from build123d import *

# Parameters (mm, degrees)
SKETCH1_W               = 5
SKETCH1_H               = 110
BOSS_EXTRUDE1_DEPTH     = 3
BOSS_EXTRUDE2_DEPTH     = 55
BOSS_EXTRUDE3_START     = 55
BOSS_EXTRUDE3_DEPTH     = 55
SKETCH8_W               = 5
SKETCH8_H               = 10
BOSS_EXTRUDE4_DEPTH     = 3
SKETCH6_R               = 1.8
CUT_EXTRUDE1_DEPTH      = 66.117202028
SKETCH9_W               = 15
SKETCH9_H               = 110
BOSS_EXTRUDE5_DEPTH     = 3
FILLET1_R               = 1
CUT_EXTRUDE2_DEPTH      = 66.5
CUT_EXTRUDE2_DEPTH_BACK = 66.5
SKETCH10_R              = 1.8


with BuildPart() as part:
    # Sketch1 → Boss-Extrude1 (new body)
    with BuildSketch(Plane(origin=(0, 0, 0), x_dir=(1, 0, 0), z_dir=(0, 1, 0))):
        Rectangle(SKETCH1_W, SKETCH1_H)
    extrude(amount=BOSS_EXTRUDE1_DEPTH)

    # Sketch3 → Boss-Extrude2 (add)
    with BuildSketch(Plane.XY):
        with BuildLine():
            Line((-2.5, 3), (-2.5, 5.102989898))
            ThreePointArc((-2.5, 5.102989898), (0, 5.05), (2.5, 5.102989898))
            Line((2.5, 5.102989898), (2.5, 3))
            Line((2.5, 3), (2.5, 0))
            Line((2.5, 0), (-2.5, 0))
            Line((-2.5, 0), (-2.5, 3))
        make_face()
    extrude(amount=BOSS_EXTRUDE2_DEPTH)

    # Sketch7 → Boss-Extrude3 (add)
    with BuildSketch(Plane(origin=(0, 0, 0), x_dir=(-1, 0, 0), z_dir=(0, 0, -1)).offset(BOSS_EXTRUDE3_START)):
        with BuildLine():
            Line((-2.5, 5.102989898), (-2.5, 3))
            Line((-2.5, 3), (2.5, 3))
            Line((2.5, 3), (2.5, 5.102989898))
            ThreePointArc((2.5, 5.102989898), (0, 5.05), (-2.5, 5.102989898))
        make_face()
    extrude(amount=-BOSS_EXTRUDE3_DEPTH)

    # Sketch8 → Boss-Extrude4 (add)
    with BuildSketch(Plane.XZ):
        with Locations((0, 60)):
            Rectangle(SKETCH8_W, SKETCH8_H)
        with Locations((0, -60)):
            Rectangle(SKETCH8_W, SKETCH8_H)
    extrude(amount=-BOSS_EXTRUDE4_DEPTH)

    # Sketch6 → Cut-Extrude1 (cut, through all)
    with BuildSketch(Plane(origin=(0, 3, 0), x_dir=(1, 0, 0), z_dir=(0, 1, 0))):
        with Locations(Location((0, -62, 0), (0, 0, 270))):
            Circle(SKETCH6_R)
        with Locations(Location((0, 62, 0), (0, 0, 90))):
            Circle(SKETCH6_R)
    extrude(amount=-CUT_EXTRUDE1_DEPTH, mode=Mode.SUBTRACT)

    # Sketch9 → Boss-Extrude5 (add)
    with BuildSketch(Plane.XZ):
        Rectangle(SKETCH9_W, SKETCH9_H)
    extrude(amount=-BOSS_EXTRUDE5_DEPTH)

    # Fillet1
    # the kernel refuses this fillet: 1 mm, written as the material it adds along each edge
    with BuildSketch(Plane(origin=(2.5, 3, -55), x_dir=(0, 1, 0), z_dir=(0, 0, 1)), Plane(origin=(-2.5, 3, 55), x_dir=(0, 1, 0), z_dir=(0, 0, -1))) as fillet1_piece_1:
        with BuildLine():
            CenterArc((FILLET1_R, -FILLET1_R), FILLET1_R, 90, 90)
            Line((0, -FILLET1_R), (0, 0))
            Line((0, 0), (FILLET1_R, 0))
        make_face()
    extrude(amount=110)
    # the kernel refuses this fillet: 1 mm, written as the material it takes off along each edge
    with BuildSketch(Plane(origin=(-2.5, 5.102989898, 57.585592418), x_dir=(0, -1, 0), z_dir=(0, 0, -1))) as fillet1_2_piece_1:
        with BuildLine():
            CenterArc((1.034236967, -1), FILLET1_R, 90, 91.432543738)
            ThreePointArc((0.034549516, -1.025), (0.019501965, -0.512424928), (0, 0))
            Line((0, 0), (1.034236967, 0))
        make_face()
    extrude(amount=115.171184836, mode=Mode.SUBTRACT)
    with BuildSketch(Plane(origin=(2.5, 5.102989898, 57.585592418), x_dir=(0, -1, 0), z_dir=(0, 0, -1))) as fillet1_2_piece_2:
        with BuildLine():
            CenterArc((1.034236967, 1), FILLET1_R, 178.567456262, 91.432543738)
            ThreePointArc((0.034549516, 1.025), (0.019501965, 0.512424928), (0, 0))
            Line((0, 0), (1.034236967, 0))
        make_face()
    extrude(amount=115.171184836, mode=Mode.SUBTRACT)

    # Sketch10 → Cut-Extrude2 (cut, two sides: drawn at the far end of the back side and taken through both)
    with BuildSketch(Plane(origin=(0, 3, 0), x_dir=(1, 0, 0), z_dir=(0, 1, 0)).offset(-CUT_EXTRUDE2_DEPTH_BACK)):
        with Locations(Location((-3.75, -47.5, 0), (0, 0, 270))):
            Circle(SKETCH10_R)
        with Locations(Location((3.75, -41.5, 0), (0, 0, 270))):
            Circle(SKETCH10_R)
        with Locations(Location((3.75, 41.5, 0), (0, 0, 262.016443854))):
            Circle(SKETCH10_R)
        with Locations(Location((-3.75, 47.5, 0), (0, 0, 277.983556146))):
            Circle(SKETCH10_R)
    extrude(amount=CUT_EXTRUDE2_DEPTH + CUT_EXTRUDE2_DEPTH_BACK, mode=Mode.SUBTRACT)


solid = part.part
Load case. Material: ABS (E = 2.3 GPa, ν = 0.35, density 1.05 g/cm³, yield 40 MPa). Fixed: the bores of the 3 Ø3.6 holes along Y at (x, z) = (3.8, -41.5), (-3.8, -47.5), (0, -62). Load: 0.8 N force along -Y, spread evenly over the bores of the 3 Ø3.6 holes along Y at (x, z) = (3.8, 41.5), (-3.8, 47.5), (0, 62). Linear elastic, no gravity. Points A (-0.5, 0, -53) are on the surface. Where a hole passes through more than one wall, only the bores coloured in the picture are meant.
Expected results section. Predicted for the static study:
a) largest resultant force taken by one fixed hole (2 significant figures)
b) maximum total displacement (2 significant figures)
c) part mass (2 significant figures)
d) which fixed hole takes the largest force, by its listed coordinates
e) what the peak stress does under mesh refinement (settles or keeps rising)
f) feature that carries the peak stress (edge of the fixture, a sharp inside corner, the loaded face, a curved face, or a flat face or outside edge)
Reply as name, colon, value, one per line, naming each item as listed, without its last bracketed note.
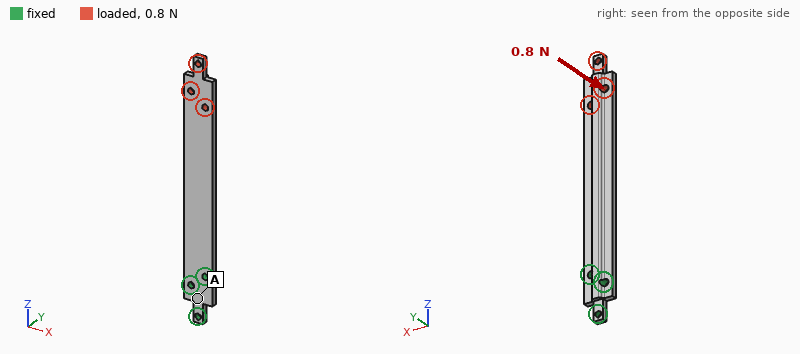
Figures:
largest resultant force taken by one fixed hole: 4.1 N
maximum total displacement: 1.3 mm
part mass: 6.5 g
which fixed hole takes the largest force, by its listed coordinates: (3.8, -41.5)
what the peak stress does under mesh refinement: keeps rising
feature that carries the peak stress: edge of the fixture
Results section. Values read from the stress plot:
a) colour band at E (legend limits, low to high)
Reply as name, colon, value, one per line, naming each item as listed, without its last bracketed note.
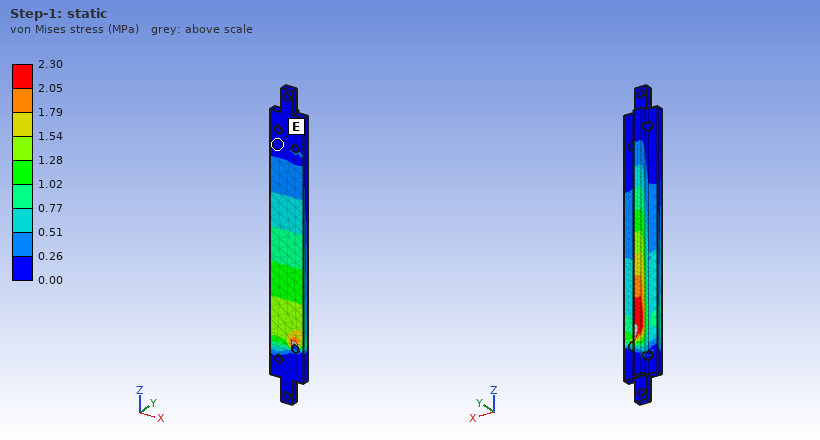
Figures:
colour band at E: 0.00 to 0.26 MPa
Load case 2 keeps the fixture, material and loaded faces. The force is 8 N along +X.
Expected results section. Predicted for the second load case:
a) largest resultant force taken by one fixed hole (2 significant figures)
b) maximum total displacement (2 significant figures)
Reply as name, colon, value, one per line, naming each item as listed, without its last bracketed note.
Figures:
largest resultant force taken by one fixed hole: 69 N
maximum total displacement: 1.4 mm
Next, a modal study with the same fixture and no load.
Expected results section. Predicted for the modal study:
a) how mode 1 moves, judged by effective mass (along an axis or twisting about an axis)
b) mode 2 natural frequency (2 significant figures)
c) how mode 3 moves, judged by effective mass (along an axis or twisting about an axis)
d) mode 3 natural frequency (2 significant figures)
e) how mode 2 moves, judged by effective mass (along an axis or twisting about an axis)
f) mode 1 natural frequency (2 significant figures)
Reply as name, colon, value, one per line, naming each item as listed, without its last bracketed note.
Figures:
how mode 1 moves, judged by effective mass: along Y
mode 2 natural frequency: 320 Hz
how mode 3 moves, judged by effective mass: along Y
mode 3 natural frequency: 650 Hz
how mode 2 moves, judged by effective mass: along X
mode 1 natural frequency: 110 Hz
